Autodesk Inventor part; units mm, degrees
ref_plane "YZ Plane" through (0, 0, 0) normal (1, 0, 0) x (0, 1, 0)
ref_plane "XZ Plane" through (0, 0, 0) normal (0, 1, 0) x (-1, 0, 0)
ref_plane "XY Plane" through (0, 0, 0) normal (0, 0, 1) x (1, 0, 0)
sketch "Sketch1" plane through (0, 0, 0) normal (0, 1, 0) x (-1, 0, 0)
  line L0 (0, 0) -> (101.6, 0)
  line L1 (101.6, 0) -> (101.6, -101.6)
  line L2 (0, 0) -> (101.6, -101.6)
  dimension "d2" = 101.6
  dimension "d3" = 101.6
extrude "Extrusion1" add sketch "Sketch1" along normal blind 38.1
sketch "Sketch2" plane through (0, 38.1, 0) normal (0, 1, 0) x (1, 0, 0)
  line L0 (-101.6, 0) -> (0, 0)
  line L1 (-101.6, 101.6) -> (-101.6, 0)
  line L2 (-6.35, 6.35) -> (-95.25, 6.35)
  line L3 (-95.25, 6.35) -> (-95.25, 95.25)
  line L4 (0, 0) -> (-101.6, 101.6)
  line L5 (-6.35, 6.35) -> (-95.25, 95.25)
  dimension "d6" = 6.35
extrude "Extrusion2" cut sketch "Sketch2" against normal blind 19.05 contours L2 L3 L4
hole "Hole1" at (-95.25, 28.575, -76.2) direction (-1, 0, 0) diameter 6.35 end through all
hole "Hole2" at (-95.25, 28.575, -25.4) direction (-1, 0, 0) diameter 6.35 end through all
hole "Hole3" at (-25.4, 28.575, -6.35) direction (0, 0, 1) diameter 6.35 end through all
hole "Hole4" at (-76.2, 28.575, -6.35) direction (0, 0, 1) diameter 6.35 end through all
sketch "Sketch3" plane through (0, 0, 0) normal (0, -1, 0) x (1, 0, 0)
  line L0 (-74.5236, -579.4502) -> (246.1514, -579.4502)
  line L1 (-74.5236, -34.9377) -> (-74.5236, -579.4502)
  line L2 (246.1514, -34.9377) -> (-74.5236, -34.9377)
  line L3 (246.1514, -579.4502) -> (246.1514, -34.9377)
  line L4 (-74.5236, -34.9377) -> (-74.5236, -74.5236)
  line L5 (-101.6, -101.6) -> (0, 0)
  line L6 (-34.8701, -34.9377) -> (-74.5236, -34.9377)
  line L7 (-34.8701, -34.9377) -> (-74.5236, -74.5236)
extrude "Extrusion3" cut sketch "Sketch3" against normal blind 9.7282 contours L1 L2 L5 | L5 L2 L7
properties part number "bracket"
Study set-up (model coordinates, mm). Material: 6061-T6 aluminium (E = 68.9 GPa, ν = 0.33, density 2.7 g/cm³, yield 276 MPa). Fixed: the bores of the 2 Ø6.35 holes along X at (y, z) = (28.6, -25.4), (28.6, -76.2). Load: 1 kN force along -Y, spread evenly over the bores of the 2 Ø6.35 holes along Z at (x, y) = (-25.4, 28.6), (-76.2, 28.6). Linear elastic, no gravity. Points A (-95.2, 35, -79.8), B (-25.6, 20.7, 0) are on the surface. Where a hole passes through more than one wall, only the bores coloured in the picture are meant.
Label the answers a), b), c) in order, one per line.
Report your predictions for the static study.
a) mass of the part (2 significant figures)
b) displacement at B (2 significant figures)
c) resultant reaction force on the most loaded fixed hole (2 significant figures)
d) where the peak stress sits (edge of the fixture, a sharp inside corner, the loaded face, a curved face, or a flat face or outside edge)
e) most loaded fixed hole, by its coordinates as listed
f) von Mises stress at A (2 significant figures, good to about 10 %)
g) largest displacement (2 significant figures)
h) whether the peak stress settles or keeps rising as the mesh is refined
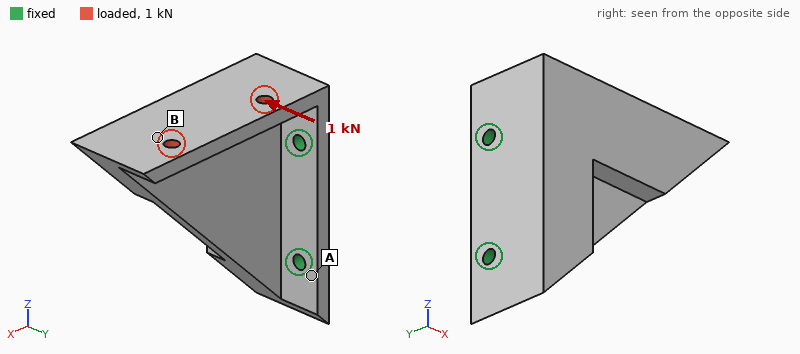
a) 300 g
b) 0.39 mm
c) 1.4 kN
d) edge of the fixture
e) (28.6, -25.4)
f) 32 MPa
g) 0.54 mm
h) keeps rising
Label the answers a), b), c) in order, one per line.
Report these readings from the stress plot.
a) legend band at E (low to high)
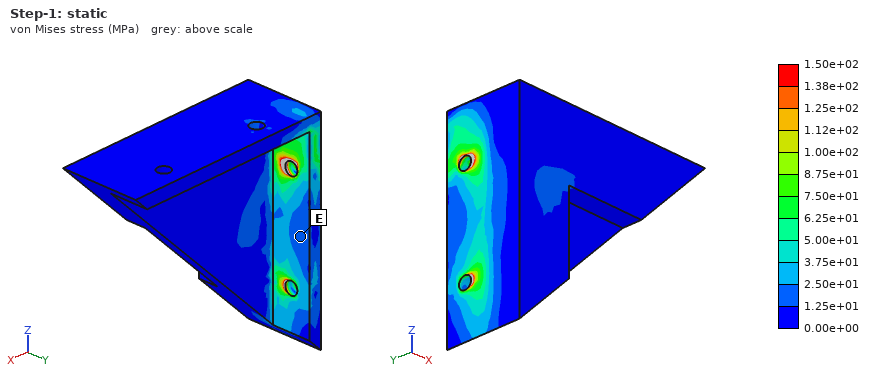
a) 1.25e+01 to 2.50e+01 MPa
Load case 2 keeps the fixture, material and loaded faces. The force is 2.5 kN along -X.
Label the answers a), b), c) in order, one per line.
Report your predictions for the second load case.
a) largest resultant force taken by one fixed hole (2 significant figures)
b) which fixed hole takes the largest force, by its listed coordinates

a) 3.3 kN
b) (28.6, -25.4)
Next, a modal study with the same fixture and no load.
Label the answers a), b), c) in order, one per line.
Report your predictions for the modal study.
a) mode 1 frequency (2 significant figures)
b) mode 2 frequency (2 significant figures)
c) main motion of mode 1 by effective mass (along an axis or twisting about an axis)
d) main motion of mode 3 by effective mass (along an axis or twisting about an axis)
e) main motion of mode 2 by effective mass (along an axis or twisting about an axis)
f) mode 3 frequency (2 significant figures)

a) 670 Hz
b) 2200 Hz
c) along Y
d) along X
e) along Z
f) 4000 Hz
